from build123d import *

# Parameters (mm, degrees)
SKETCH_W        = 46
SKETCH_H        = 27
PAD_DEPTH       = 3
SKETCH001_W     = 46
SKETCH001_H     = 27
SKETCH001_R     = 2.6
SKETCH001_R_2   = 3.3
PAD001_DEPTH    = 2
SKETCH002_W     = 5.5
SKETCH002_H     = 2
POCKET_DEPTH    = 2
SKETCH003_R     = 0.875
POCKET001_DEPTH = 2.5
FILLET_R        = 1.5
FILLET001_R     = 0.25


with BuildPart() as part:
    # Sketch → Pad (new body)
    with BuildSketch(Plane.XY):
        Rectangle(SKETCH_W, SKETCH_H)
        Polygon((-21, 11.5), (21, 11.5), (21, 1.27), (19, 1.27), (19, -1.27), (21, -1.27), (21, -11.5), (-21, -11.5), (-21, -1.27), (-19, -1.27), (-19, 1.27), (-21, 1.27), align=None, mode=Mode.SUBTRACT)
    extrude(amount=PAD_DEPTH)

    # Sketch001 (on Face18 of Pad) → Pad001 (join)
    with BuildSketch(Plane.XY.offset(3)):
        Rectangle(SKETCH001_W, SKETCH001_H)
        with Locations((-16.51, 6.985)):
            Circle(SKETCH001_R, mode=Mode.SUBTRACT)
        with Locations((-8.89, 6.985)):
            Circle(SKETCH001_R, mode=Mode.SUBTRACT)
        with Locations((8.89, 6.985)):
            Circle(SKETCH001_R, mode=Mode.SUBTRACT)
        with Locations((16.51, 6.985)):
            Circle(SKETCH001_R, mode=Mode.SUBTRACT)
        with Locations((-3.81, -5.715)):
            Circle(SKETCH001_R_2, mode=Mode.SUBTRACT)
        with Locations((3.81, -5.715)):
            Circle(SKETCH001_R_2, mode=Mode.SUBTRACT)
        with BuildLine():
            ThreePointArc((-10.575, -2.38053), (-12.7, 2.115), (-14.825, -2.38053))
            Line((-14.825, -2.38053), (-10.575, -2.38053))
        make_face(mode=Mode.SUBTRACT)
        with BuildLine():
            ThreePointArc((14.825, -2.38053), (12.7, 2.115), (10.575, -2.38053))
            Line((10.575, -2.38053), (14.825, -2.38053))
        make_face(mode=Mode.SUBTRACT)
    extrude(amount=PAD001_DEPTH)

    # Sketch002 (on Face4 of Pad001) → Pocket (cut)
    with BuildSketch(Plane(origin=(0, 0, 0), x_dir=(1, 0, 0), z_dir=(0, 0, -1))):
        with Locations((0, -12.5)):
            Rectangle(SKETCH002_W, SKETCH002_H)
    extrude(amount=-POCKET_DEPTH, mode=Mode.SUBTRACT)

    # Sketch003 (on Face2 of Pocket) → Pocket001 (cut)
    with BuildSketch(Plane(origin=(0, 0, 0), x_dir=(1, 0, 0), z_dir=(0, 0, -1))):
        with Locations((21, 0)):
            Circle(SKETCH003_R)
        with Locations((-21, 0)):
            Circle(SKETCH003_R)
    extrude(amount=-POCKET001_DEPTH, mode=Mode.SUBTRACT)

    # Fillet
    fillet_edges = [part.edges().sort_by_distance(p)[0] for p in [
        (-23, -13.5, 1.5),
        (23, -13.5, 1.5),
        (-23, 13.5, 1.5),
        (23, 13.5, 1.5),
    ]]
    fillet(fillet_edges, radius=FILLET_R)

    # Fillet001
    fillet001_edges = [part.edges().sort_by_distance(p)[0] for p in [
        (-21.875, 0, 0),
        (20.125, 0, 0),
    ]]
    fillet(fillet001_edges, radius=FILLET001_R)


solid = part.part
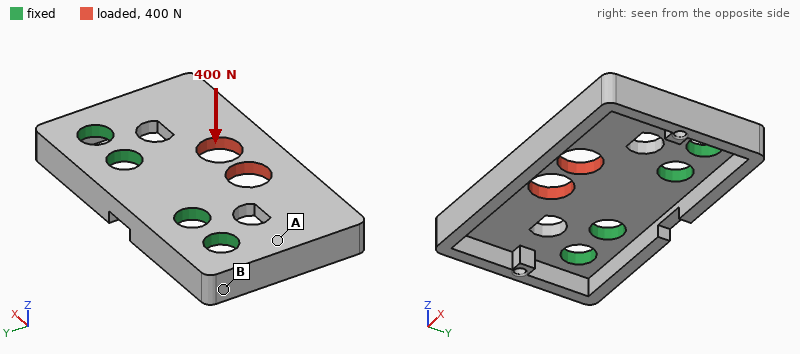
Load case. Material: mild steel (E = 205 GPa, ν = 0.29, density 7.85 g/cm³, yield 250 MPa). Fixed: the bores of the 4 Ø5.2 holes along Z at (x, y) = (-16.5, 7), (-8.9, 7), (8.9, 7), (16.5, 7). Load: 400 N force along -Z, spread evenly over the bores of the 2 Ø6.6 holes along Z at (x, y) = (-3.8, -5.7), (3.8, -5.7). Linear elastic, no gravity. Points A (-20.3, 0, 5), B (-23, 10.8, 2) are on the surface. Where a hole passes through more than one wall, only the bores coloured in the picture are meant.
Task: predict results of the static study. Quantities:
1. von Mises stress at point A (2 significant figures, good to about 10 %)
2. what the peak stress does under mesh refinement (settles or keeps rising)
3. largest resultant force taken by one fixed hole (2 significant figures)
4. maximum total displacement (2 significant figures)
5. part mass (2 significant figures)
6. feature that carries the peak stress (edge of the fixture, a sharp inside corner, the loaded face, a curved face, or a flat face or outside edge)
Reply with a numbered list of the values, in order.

1. 51 MPa
2. keeps rising
3. 160 N
4. 49 µm
5. 23 g
6. edge of the fixture
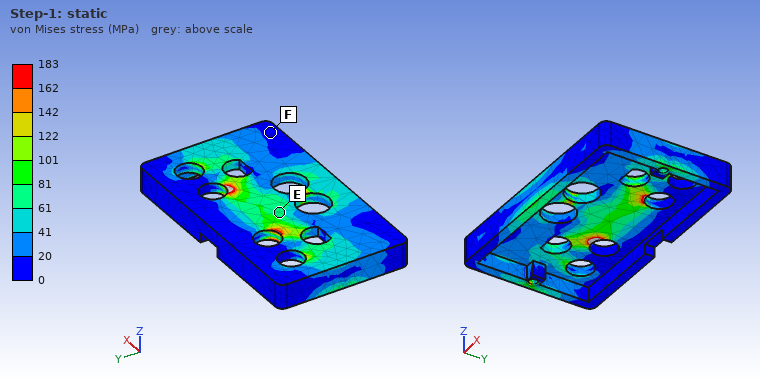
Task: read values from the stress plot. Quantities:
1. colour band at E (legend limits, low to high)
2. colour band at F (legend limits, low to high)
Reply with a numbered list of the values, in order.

1. 61 to 81 MPa
2. 0 to 20 MPa
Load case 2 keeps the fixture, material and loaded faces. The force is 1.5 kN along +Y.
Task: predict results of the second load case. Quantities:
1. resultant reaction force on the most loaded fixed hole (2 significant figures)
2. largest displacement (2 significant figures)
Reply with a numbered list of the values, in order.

1. 650 N
2. 5.2 µm
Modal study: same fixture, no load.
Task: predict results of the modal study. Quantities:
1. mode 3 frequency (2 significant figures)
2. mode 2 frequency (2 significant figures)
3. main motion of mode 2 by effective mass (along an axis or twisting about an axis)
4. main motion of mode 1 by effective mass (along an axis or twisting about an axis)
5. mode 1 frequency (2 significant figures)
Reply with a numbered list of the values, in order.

1. 13 kHz
2. 6300 Hz
3. twisting about Y
4. along Z
5. 4500 Hz
